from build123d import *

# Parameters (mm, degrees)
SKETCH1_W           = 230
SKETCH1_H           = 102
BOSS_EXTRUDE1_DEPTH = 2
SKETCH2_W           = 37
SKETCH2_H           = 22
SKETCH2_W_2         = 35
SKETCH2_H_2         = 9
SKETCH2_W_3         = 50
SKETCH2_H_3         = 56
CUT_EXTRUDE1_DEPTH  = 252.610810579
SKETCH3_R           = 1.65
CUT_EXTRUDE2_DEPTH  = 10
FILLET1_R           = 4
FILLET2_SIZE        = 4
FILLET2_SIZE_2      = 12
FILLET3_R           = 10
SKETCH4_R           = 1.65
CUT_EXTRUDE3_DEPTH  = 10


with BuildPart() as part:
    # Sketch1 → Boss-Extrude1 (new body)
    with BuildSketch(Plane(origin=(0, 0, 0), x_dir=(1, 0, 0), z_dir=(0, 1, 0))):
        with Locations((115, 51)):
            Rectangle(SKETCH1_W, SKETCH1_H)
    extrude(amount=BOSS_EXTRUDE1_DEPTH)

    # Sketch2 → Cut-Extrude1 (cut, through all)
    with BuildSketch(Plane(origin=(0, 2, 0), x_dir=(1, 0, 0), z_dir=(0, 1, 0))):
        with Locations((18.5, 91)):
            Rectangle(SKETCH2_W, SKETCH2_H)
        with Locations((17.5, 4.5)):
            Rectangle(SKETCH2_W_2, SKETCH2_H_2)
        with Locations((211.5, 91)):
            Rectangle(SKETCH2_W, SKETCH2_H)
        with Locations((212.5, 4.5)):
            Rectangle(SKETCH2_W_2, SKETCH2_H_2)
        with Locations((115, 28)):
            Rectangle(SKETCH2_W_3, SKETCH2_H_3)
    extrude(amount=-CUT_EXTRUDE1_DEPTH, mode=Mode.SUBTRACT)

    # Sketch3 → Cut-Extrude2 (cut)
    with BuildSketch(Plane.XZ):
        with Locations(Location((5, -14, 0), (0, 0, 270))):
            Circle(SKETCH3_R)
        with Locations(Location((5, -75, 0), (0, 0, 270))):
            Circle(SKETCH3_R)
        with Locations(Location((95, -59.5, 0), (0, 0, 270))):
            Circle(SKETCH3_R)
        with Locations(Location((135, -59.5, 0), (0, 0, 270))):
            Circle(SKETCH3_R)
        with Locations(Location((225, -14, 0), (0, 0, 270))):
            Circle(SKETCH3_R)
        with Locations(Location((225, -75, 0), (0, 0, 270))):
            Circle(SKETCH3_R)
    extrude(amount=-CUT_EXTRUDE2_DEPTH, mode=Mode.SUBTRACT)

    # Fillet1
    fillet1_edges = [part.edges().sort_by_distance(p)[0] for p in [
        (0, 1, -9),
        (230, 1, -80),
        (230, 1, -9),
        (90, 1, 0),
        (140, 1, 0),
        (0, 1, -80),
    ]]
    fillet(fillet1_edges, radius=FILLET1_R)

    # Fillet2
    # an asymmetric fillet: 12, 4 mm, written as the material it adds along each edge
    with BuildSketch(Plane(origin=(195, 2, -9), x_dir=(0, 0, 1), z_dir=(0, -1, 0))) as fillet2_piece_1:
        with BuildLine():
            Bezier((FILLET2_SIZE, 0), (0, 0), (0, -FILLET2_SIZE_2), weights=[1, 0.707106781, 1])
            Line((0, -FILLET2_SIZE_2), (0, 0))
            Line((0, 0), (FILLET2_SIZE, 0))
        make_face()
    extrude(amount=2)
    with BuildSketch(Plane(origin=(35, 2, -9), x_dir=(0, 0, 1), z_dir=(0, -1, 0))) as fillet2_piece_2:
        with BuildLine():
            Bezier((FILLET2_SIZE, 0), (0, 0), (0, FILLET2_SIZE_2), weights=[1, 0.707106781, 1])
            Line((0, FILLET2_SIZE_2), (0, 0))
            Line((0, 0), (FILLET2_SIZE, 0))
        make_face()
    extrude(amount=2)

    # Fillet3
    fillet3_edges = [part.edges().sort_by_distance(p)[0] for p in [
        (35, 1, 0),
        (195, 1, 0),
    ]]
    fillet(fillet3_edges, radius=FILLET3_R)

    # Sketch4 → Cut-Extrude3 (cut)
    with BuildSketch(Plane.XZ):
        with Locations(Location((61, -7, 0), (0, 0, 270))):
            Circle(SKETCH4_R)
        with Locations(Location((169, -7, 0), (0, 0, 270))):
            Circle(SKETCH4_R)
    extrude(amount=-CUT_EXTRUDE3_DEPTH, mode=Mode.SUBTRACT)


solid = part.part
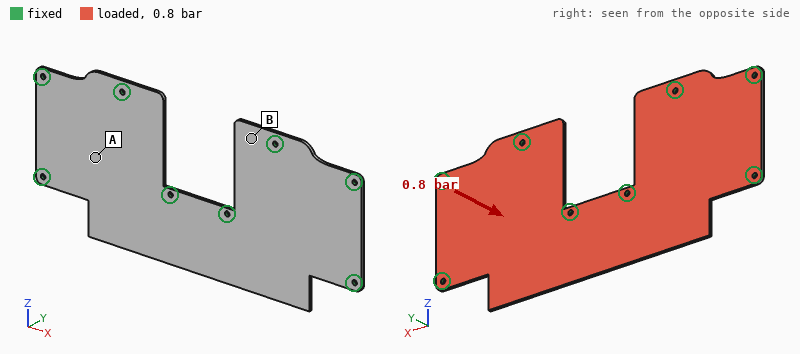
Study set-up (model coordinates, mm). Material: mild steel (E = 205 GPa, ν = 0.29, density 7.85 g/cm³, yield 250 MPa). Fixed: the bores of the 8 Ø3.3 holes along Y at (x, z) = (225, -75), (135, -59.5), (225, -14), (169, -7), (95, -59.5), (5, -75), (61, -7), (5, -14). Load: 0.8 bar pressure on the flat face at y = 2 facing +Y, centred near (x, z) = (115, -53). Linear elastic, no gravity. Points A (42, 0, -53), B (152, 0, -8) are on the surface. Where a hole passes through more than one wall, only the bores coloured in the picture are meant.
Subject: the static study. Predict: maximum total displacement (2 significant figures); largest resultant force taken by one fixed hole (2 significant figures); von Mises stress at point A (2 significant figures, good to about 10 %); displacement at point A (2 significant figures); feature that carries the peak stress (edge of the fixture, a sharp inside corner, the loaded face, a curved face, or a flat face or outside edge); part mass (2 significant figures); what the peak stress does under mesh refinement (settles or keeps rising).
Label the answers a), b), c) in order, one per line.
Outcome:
a) 0.40 mm
b) 310 N
c) 40 MPa
d) 0.12 mm
e) edge of the fixture
f) 290 g
g) keeps rising
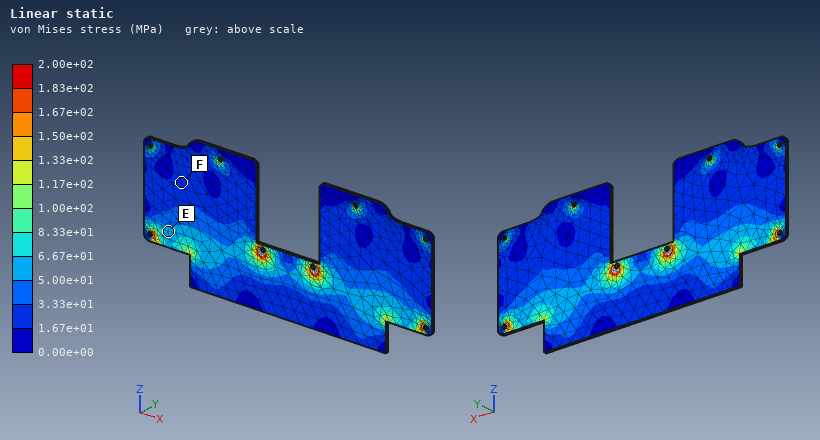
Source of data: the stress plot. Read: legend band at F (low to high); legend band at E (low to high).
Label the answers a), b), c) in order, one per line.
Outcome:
a) 1.67e+01 to 3.33e+01 MPa
b) 5.00e+01 to 6.67e+01 MPa
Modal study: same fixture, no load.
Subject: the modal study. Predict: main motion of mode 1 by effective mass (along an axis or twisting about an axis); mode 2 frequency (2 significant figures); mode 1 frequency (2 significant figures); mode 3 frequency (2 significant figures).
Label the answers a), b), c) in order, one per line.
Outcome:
a) along Y
b) 830 Hz
c) 730 Hz
d) 1200 Hz
